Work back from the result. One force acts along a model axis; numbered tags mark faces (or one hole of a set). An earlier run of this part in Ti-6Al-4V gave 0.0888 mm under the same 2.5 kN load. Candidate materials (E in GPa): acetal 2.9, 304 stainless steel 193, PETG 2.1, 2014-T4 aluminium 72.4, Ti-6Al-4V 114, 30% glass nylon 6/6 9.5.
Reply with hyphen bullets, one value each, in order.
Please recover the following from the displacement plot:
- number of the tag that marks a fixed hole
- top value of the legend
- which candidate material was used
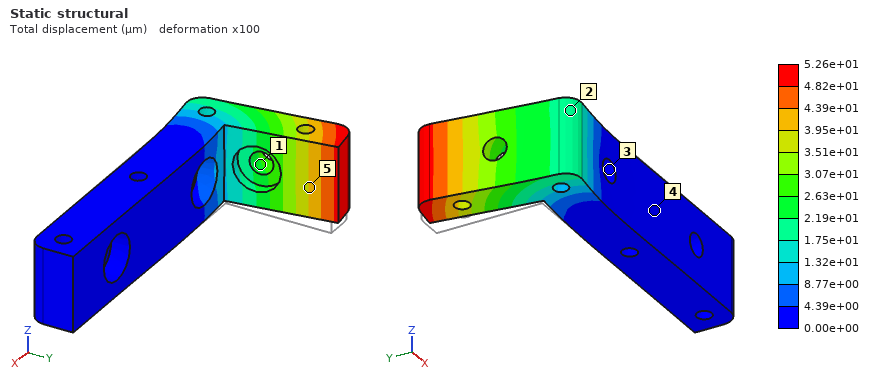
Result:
- 3
- 5.26e+01 µm
- 304 stainless steel
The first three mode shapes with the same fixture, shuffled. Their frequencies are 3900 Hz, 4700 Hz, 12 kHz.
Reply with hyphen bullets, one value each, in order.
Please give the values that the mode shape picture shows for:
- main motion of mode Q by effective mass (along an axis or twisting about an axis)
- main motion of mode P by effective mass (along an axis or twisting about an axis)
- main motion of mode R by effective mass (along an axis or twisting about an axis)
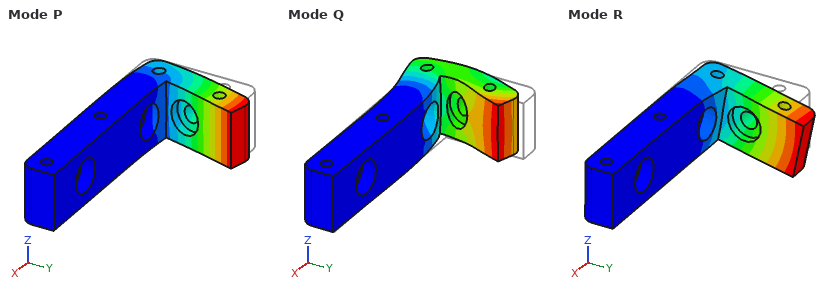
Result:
- along Y
- along X
- along Z
